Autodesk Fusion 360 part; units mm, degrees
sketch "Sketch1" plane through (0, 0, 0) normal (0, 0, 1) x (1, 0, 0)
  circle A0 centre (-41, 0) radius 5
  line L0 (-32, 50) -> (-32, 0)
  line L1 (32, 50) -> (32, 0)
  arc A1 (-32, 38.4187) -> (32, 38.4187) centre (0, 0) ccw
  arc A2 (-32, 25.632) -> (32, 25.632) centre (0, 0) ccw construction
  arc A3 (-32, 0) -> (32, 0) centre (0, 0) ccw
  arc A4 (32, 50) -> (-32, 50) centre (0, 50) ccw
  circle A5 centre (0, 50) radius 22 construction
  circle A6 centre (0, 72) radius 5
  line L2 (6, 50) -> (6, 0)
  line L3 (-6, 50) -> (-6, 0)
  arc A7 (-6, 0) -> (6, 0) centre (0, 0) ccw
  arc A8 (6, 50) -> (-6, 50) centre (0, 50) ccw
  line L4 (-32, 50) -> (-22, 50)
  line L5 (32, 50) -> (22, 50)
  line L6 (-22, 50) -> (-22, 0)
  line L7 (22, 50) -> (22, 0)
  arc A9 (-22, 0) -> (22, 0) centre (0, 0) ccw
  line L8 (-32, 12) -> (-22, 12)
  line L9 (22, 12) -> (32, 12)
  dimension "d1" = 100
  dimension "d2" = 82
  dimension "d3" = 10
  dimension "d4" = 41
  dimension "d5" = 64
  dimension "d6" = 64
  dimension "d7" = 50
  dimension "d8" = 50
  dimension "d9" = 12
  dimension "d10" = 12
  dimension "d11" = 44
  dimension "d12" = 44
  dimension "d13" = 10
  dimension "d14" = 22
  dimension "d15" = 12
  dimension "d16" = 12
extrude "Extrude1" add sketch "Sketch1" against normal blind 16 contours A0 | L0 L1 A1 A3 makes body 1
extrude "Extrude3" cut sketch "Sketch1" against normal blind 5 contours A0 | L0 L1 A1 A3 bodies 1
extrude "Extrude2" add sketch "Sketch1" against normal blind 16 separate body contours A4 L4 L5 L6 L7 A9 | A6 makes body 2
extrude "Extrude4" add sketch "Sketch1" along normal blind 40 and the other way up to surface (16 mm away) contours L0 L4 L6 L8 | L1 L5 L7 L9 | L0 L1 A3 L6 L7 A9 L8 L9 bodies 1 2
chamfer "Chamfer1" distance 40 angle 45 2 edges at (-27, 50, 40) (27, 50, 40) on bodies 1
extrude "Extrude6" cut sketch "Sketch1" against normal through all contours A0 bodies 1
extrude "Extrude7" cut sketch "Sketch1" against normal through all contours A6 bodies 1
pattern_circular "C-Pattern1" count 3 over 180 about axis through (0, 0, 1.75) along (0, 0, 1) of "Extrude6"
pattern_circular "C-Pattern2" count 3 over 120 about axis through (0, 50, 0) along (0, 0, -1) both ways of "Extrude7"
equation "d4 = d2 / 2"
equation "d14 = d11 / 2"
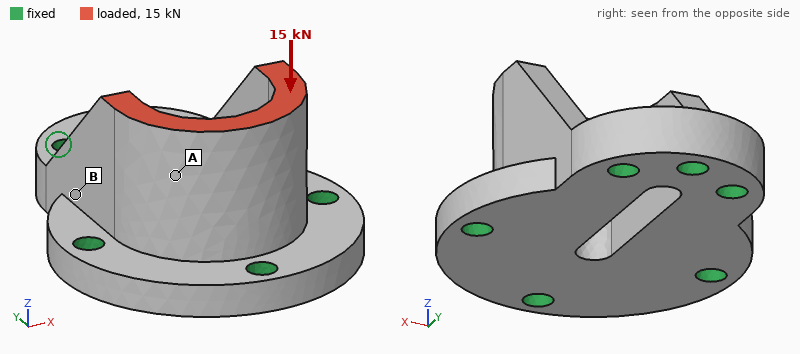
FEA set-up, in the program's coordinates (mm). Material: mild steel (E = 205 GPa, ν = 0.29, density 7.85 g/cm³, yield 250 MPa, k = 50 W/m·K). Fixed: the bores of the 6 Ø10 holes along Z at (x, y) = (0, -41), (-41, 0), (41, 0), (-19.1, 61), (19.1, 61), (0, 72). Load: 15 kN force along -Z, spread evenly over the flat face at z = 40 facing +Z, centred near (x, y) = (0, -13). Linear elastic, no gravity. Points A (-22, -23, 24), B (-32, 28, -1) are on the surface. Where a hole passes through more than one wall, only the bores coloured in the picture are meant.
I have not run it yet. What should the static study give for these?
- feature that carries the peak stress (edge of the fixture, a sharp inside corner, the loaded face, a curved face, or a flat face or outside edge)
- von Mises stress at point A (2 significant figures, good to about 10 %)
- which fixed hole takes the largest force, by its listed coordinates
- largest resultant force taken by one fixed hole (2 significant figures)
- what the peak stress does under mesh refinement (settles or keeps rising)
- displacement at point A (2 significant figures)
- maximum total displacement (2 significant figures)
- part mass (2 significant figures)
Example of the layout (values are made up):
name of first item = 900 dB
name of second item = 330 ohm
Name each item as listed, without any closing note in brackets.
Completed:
feature that carries the peak stress = edge of the fixture
von Mises stress at point A = 15 MPa
which fixed hole takes the largest force, by its listed coordinates = (0, -41)
largest resultant force taken by one fixed hole = 6.5 kN
what the peak stress does under mesh refinement = keeps rising
displacement at point A = 7.1 µm
maximum total displacement = 9.2 µm
part mass = 1.4 kg
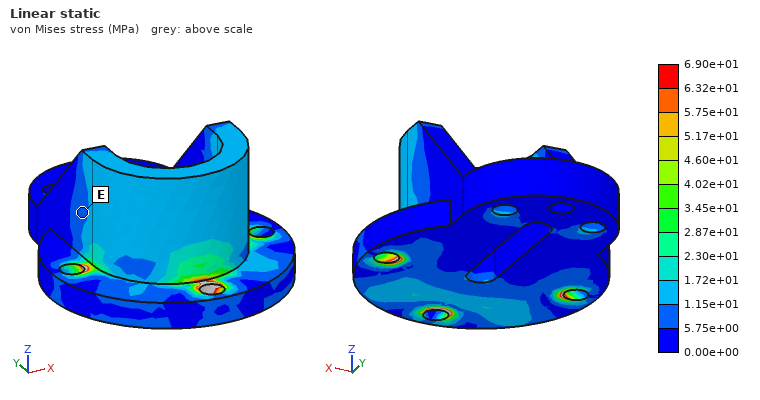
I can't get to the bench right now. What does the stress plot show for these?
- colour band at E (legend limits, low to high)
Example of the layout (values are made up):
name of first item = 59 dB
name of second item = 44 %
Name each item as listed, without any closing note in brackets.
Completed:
colour band at E = 5.75e+00 to 1.15e+01 MPa
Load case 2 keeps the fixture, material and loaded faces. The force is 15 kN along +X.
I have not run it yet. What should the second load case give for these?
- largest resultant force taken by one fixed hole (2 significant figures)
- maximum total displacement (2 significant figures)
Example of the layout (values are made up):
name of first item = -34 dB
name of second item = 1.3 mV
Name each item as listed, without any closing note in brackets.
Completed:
largest resultant force taken by one fixed hole = 12 kN
maximum total displacement = 70 µm
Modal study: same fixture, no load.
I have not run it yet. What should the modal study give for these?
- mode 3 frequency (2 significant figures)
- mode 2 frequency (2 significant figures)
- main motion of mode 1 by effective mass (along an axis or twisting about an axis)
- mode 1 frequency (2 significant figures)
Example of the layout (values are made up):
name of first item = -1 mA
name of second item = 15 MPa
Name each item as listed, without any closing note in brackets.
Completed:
mode 3 frequency = 9900 Hz
mode 2 frequency = 7400 Hz
main motion of mode 1 by effective mass = along X
mode 1 frequency = 6500 Hz
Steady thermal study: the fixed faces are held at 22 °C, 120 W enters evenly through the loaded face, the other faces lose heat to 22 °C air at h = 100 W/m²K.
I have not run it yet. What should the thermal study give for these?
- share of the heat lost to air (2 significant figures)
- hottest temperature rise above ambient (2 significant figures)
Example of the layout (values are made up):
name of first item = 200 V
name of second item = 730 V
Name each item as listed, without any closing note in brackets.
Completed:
share of the heat lost to air = 49 %
hottest temperature rise above ambient = 84 K
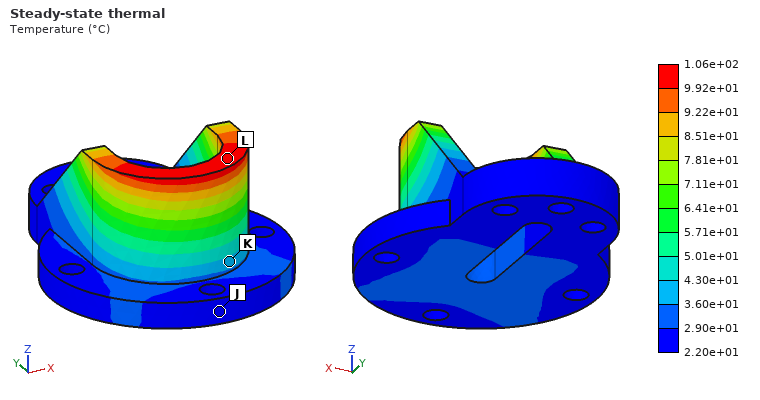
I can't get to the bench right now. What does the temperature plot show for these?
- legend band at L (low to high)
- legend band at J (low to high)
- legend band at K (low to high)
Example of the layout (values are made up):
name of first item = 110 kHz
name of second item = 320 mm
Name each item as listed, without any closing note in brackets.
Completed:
legend band at L = 9.92e+01 to 1.06e+02 °C
legend band at J = 2.20e+01 to 2.90e+01 °C
legend band at K = 3.60e+01 to 4.30e+01 °C
